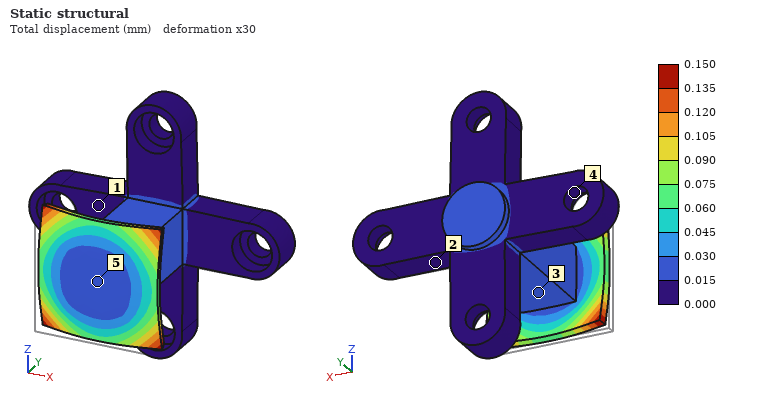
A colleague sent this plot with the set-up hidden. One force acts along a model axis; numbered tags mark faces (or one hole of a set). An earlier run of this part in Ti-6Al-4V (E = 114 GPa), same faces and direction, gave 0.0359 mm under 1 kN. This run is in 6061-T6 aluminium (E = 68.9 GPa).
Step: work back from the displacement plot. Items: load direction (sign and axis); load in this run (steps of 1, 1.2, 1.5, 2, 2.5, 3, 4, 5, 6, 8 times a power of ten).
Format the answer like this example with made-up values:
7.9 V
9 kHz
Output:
+Y
2.5 kN
